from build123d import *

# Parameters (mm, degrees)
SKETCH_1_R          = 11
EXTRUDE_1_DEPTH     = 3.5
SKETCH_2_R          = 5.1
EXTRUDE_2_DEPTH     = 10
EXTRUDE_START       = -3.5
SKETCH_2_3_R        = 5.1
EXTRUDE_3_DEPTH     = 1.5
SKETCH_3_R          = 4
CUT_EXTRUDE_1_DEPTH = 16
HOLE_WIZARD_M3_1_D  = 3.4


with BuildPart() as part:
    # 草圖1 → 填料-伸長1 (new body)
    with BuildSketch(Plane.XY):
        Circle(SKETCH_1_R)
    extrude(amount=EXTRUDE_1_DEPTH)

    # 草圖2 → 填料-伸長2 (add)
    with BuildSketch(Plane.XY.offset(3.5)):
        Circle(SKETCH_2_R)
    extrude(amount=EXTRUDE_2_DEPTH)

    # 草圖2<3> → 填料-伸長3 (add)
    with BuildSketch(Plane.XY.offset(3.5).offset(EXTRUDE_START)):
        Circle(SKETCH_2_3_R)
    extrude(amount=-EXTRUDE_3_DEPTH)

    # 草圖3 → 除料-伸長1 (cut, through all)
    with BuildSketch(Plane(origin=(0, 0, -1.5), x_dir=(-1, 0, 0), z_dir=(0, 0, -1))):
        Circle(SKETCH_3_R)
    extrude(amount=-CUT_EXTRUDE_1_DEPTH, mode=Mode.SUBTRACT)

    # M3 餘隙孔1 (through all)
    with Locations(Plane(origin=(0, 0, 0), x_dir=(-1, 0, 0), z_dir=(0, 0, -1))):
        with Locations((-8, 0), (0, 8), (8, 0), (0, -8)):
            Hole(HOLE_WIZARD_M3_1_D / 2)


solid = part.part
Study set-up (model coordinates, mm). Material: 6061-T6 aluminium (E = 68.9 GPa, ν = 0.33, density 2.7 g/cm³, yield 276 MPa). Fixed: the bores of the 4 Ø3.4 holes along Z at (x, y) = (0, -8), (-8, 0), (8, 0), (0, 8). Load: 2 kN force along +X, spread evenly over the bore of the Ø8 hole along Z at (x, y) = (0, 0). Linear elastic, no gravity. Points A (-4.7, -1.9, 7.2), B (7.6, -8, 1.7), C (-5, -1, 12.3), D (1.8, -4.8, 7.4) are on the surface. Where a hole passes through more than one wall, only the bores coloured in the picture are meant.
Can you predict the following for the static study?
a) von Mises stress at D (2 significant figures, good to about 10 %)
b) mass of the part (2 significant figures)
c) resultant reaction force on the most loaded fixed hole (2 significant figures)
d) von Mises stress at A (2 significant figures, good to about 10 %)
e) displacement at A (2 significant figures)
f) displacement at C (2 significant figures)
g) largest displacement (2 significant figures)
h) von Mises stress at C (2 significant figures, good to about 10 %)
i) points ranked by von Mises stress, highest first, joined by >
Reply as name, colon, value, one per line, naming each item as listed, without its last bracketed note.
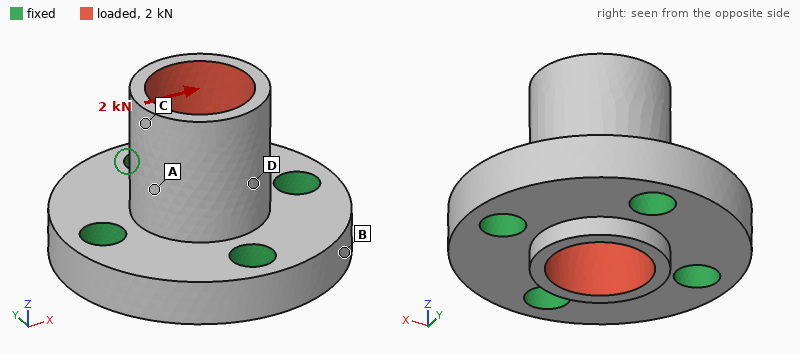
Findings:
von Mises stress at D: 74 MPa
mass of the part: 3.8 g
resultant reaction force on the most loaded fixed hole: 830 N
von Mises stress at A: 42 MPa
displacement at A: 18 µm
displacement at C: 32 µm
largest displacement: 35 µm
von Mises stress at C: 22 MPa
points ranked by von Mises stress, highest first, joined by >: D > A > C > B
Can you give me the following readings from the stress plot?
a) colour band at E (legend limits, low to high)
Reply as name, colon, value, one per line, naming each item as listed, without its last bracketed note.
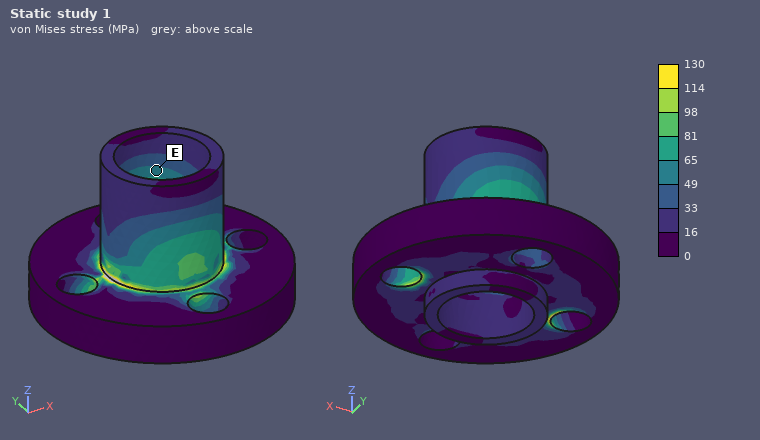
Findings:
colour band at E: 49 to 65 MPa
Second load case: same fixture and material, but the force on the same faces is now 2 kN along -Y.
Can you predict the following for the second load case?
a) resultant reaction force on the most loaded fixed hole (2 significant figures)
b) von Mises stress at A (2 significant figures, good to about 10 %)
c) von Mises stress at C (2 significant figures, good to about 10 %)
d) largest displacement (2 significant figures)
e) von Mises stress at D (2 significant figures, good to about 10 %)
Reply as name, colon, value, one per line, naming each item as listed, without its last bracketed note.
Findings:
resultant reaction force on the most loaded fixed hole: 830 N
von Mises stress at A: 75 MPa
von Mises stress at C: 16 MPa
largest displacement: 35 µm
von Mises stress at D: 41 MPa
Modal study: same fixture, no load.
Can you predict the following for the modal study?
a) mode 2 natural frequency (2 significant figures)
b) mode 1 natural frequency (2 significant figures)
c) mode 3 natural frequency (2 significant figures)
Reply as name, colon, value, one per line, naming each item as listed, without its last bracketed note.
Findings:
mode 2 natural frequency: 39 kHz
mode 1 natural frequency: 39 kHz
mode 3 natural frequency: 42 kHz
